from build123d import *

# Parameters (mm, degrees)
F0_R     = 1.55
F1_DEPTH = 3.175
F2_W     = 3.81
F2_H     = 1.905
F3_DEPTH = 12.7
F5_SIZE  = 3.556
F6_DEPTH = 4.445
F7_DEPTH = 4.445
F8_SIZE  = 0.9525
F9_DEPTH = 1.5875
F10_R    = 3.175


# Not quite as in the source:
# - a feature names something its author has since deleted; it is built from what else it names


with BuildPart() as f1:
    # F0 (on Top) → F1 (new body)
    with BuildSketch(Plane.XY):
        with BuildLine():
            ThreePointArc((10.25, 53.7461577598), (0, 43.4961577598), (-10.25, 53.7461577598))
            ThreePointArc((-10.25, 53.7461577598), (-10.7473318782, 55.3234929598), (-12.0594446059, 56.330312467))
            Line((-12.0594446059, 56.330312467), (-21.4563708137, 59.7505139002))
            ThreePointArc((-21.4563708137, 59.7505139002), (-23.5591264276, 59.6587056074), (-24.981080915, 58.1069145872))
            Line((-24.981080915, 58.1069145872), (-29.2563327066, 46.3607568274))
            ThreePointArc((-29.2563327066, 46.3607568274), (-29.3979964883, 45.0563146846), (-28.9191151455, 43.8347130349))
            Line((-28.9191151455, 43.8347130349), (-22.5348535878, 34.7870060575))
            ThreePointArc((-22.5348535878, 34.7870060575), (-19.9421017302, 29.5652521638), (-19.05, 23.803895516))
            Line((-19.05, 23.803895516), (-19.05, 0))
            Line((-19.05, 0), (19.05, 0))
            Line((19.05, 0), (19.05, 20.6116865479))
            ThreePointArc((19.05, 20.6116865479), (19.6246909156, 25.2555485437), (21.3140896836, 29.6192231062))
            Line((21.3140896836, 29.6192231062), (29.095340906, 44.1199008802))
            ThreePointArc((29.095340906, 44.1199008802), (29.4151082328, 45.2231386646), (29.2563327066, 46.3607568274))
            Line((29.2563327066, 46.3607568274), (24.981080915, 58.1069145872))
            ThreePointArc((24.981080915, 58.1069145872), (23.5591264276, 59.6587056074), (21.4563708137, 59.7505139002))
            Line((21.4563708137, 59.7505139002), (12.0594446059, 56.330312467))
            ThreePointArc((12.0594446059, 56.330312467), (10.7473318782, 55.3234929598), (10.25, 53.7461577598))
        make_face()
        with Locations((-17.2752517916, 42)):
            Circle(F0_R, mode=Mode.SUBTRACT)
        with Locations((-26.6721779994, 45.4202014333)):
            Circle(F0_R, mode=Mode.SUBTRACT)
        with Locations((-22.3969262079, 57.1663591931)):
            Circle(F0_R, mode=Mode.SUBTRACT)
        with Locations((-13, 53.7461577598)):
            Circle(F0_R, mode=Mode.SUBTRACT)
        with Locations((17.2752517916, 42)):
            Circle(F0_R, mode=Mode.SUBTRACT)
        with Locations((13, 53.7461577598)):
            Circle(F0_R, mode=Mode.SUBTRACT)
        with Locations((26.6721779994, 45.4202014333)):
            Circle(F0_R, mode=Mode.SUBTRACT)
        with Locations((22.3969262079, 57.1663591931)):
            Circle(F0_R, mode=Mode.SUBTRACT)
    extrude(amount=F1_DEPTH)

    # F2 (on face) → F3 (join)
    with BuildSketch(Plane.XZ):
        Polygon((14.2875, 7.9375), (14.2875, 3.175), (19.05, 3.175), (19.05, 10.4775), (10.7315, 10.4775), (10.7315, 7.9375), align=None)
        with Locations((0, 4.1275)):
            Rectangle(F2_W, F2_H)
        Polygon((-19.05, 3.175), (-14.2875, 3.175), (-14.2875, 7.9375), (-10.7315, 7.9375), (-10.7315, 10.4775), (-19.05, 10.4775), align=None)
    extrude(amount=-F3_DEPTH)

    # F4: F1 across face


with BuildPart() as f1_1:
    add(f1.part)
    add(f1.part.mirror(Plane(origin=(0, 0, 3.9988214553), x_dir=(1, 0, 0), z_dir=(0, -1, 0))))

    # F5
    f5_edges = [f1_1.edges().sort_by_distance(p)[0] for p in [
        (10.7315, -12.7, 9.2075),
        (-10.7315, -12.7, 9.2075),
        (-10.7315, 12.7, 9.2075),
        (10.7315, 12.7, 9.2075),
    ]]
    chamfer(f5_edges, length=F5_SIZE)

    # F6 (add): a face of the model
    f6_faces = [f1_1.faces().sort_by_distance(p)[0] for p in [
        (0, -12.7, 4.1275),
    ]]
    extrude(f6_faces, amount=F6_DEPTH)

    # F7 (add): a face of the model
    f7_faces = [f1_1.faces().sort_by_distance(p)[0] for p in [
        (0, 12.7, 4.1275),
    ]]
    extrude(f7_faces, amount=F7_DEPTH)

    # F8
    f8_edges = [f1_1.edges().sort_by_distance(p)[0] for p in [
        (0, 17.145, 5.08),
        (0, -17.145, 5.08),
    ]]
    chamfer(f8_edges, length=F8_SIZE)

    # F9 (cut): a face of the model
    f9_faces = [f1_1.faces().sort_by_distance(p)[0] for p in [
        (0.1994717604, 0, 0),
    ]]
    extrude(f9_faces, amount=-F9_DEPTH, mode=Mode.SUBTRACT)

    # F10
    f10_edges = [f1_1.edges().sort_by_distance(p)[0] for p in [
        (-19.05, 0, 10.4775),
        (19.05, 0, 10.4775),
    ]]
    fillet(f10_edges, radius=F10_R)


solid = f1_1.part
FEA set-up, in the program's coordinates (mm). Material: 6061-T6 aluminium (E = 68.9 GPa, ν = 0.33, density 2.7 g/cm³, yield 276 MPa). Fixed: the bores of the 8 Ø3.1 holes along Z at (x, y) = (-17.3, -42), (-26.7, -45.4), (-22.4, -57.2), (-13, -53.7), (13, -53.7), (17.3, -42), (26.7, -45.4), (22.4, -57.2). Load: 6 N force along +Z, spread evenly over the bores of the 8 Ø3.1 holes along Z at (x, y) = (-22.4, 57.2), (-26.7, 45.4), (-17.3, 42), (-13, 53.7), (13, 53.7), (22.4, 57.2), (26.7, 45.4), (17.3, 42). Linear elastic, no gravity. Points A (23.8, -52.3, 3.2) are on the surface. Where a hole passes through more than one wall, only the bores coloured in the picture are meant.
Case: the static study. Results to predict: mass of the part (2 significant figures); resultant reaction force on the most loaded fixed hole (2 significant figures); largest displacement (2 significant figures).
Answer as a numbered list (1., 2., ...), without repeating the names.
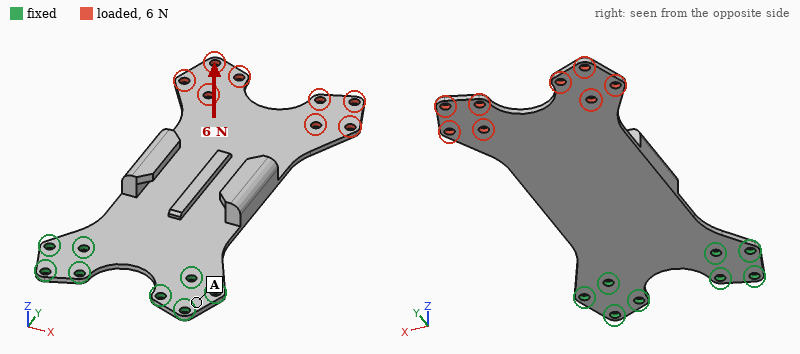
1. 26 g
2. 20 N
3. 1.5 mm
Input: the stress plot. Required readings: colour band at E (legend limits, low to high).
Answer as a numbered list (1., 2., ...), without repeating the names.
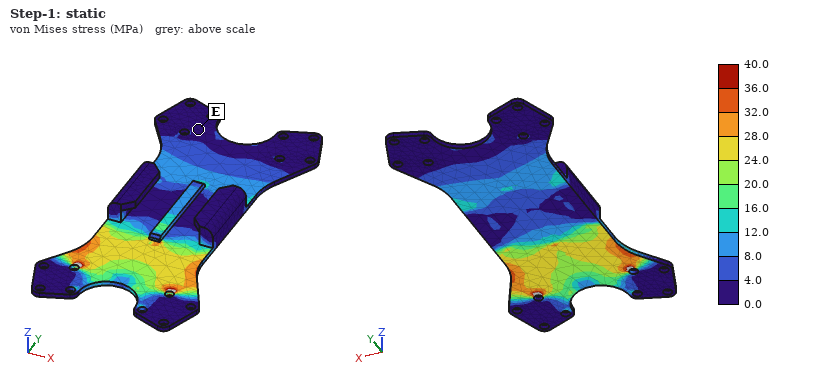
1. 0.0 to 4.0 MPa
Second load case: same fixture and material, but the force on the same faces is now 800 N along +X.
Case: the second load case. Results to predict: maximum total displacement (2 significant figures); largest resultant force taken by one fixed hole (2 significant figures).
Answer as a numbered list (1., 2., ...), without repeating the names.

1. 0.47 mm
2. 1.4 kN
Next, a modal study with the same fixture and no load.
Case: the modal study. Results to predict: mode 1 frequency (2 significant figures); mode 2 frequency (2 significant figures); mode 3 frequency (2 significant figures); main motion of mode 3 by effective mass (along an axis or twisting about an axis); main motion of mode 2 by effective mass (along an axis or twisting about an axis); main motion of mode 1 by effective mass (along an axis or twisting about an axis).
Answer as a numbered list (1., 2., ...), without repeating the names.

1. 140 Hz
2. 590 Hz
3. 910 Hz
4. along Z
5. twisting about Y
6. along Z
